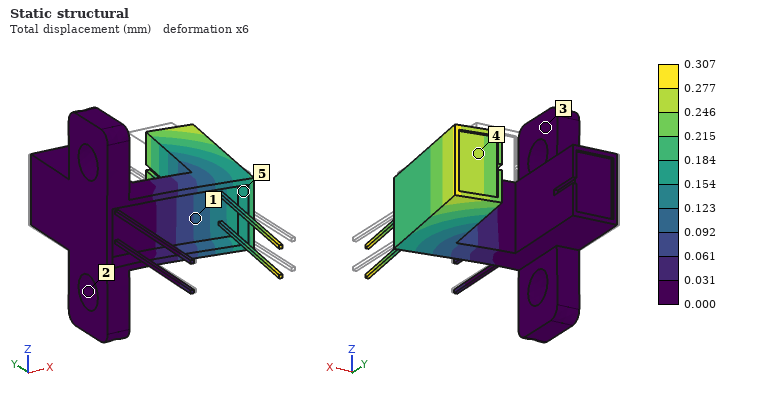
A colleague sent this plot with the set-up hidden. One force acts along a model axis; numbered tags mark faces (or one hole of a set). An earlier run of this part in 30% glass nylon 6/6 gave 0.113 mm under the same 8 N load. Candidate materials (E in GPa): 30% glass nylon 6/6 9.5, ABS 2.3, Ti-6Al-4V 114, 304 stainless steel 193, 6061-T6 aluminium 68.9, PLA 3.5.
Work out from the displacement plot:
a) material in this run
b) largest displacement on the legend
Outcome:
PLA
0.307 mm
